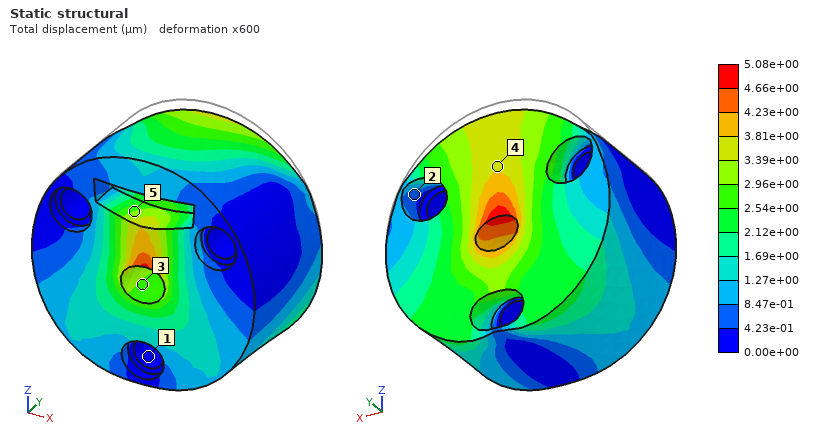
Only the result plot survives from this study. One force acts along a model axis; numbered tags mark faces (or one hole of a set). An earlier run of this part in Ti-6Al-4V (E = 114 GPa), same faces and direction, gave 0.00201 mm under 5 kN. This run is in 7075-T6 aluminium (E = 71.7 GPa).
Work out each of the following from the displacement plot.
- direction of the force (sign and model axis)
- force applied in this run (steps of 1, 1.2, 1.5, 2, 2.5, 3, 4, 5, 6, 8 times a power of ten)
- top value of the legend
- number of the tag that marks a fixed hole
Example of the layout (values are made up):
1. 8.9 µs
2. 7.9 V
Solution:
1. -Z
2. 8 kN
3. 5.08e+00 µm
4. 1
